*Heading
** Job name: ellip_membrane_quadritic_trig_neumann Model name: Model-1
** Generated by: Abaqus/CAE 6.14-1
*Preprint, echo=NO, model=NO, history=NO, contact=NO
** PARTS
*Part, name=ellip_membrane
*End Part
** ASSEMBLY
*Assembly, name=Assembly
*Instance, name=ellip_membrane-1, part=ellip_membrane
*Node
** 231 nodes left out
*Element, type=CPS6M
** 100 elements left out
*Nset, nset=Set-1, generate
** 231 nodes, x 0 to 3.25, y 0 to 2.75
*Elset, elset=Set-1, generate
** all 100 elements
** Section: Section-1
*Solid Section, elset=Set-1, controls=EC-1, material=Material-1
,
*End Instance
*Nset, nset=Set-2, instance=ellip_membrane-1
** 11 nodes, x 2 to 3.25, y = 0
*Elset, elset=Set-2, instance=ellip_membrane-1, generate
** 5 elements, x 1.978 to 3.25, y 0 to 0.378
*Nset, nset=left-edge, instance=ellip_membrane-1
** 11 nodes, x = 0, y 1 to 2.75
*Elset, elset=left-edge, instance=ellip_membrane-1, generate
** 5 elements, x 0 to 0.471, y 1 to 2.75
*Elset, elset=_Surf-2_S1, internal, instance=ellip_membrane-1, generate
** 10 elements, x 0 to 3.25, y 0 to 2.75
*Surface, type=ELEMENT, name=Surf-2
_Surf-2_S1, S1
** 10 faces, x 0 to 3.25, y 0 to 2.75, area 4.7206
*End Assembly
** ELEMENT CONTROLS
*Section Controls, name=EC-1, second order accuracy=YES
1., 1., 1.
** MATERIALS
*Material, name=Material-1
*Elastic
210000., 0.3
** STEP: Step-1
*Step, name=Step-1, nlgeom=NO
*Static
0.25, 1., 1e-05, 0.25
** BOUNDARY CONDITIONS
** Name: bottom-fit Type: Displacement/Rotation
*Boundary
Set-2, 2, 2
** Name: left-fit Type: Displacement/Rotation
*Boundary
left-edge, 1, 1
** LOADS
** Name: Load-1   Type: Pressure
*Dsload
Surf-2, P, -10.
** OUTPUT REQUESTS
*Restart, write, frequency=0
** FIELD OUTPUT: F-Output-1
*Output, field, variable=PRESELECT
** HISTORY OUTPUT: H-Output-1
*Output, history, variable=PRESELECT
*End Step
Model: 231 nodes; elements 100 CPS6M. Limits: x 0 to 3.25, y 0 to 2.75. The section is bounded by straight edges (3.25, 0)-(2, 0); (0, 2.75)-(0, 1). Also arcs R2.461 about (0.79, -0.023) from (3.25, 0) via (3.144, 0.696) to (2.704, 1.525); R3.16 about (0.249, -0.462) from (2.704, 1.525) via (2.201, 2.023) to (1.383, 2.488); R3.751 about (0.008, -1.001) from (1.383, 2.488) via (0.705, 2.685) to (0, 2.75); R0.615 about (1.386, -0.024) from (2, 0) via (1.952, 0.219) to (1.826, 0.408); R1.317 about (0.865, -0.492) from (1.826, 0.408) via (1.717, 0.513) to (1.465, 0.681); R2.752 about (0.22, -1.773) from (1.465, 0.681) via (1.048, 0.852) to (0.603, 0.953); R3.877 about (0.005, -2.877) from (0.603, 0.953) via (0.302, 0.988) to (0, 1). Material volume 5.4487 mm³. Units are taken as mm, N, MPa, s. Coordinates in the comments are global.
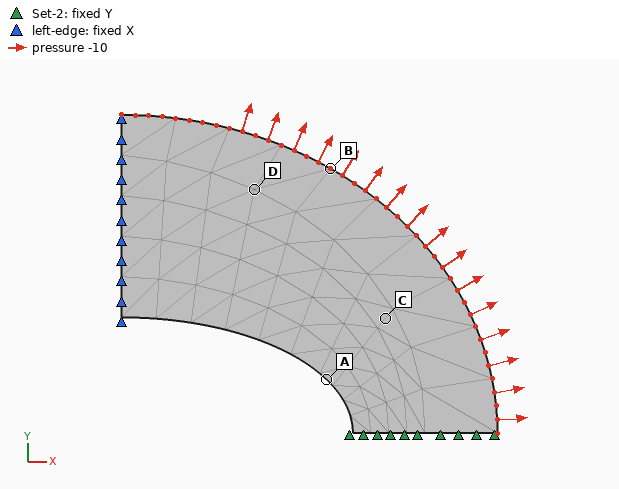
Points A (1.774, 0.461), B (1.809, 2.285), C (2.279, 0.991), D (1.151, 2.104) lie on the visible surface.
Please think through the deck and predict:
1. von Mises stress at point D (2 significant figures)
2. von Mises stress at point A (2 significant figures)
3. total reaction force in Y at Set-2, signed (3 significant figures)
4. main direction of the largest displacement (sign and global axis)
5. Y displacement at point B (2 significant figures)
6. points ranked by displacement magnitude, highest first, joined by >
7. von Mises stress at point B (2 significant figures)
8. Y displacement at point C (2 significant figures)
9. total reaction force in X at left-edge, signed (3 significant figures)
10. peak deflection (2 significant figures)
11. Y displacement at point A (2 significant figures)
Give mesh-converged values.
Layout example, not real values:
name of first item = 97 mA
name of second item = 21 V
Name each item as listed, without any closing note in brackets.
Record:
von Mises stress at point D = 21 MPa
von Mises stress at point A = 44 MPa
total reaction force in Y at Set-2, signed = -32.5 N
main direction of the largest displacement = +Y
Y displacement at point B = 3.2e-04 mm
points ranked by displacement magnitude, highest first, joined by > = D > B > A > C
von Mises stress at point B = 22 MPa
Y displacement at point C = 1.4e-04 mm
total reaction force in X at left-edge, signed = -27.5 N
peak deflection = 5.5e-04 mm
Y displacement at point A = 2.1e-04 mm
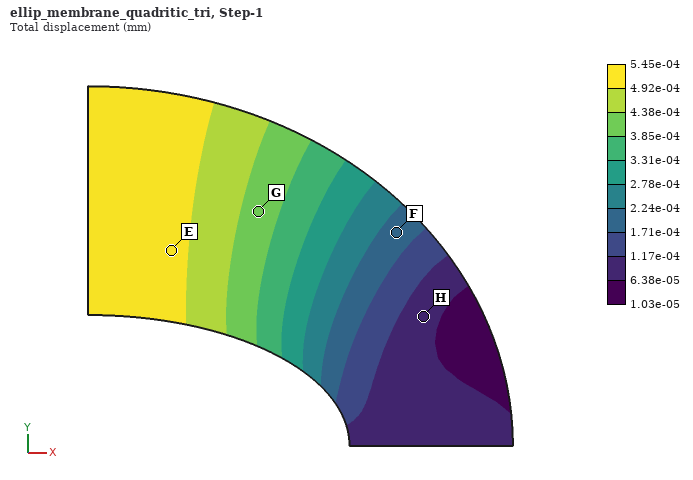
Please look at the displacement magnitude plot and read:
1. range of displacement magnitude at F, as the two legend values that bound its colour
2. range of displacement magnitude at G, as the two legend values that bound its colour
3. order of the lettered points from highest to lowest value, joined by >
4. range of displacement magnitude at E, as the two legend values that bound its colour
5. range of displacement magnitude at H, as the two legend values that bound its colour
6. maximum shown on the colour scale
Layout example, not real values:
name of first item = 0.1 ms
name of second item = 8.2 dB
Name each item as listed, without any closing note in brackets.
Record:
range of displacement magnitude at F, as the two legend values that bound its colour = 1.71e-04 to 2.24e-04 mm
range of displacement magnitude at G, as the two legend values that bound its colour = 3.85e-04 to 4.38e-04 mm
order of the lettered points from highest to lowest value, joined by > = E > G > F > H
range of displacement magnitude at E, as the two legend values that bound its colour = 4.92e-04 to 5.45e-04 mm
range of displacement magnitude at H, as the two legend values that bound its colour = 6.38e-05 to 1.17e-04 mm
maximum shown on the colour scale = 5.45e-04 mm
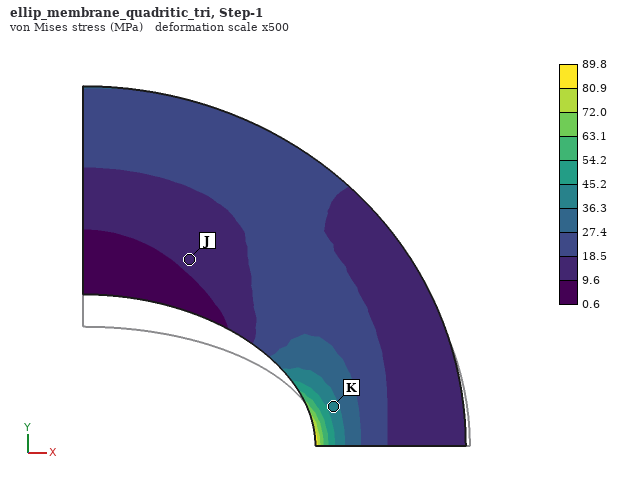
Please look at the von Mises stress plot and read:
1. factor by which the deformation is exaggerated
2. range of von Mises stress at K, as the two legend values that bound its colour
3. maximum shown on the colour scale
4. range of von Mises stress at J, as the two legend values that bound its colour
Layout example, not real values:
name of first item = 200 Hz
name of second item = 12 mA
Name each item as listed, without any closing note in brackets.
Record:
factor by which the deformation is exaggerated = 500
range of von Mises stress at K, as the two legend values that bound its colour = 36.3 to 45.2 MPa
maximum shown on the colour scale = 89.8 MPa
range of von Mises stress at J, as the two legend values that bound its colour = 9.6 to 18.5 MPa
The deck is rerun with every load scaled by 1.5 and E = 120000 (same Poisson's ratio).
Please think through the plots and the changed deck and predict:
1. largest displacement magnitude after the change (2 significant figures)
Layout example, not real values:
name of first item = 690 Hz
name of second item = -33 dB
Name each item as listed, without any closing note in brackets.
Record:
largest displacement magnitude after the change = 0.0014 mm
